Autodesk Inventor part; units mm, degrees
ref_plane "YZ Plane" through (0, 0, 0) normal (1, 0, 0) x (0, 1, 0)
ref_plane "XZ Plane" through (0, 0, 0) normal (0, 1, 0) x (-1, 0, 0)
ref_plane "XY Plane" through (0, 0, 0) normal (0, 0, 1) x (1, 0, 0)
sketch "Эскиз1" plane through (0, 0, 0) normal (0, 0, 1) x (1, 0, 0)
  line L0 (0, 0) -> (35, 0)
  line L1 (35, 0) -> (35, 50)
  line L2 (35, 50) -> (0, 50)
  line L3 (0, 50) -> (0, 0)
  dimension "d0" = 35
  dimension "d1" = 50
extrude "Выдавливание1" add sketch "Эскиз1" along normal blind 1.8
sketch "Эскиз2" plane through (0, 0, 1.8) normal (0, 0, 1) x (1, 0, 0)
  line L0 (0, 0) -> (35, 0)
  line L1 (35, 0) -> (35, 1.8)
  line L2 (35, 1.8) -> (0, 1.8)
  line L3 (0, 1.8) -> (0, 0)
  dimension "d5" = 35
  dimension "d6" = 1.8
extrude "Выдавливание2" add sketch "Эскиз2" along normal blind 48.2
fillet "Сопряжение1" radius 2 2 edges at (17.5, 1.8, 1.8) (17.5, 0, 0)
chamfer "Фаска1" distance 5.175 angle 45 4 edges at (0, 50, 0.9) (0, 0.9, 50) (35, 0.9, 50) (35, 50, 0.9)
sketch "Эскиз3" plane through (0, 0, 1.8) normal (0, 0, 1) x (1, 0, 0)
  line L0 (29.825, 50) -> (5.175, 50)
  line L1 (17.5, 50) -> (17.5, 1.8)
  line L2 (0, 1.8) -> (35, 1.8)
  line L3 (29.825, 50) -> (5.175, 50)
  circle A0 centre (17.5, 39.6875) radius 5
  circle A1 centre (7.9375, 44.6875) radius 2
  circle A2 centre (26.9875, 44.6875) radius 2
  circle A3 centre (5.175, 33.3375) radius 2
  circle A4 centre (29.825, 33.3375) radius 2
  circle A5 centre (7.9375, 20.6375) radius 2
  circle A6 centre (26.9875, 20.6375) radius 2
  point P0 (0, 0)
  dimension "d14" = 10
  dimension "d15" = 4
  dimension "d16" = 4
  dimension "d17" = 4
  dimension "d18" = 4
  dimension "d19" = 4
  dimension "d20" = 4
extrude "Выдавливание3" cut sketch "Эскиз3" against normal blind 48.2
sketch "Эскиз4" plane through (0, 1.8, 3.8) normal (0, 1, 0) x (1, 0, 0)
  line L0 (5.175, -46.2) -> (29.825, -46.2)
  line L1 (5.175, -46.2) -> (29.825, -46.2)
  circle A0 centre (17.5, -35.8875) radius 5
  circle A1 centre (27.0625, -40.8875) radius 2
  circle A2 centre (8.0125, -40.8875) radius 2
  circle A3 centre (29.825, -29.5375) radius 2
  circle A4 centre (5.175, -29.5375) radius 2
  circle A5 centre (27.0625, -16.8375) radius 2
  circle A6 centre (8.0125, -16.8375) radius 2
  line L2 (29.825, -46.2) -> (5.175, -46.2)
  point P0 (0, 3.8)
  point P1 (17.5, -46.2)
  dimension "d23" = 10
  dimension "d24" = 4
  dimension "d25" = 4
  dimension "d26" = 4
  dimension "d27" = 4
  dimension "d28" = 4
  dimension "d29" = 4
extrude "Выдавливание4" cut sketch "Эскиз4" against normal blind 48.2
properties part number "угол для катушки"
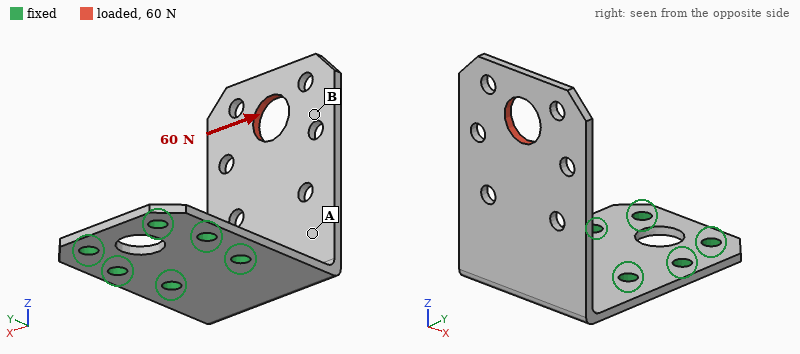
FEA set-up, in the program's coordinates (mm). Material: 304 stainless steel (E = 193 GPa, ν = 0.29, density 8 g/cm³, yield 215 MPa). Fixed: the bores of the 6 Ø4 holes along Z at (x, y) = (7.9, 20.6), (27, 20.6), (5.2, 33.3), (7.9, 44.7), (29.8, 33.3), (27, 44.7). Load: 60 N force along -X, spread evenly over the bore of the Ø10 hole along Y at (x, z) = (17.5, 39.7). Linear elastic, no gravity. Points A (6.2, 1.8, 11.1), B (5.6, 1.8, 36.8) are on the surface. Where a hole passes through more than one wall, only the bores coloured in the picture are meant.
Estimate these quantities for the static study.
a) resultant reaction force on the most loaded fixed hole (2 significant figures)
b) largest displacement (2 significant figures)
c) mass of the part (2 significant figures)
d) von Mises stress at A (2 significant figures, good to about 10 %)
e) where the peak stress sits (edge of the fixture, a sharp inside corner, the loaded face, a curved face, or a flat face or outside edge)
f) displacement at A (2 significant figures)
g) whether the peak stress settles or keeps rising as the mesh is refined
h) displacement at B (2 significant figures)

120 N
0.19 mm
44 g
23 MPa
edge of the fixture
0.058 mm
keeps rising
0.14 mm
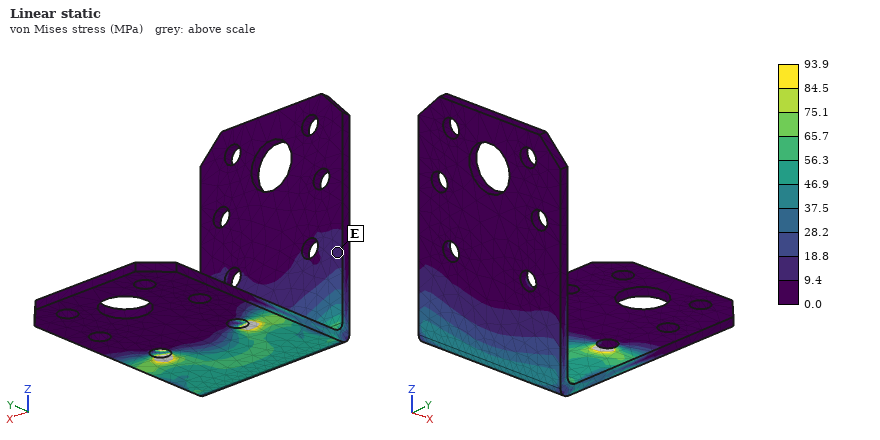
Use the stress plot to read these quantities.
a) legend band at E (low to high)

9.4 to 18.8 MPa
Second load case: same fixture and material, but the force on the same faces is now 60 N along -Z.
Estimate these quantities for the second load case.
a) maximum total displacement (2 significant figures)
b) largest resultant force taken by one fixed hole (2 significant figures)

0.16 mm
38 N
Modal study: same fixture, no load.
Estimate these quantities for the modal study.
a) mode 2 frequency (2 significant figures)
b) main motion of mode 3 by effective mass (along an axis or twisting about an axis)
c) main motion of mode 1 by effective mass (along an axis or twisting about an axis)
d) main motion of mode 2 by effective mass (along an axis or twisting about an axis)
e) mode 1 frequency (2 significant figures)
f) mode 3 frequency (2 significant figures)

910 Hz
along Z
along Y
along X
430 Hz
1700 Hz
